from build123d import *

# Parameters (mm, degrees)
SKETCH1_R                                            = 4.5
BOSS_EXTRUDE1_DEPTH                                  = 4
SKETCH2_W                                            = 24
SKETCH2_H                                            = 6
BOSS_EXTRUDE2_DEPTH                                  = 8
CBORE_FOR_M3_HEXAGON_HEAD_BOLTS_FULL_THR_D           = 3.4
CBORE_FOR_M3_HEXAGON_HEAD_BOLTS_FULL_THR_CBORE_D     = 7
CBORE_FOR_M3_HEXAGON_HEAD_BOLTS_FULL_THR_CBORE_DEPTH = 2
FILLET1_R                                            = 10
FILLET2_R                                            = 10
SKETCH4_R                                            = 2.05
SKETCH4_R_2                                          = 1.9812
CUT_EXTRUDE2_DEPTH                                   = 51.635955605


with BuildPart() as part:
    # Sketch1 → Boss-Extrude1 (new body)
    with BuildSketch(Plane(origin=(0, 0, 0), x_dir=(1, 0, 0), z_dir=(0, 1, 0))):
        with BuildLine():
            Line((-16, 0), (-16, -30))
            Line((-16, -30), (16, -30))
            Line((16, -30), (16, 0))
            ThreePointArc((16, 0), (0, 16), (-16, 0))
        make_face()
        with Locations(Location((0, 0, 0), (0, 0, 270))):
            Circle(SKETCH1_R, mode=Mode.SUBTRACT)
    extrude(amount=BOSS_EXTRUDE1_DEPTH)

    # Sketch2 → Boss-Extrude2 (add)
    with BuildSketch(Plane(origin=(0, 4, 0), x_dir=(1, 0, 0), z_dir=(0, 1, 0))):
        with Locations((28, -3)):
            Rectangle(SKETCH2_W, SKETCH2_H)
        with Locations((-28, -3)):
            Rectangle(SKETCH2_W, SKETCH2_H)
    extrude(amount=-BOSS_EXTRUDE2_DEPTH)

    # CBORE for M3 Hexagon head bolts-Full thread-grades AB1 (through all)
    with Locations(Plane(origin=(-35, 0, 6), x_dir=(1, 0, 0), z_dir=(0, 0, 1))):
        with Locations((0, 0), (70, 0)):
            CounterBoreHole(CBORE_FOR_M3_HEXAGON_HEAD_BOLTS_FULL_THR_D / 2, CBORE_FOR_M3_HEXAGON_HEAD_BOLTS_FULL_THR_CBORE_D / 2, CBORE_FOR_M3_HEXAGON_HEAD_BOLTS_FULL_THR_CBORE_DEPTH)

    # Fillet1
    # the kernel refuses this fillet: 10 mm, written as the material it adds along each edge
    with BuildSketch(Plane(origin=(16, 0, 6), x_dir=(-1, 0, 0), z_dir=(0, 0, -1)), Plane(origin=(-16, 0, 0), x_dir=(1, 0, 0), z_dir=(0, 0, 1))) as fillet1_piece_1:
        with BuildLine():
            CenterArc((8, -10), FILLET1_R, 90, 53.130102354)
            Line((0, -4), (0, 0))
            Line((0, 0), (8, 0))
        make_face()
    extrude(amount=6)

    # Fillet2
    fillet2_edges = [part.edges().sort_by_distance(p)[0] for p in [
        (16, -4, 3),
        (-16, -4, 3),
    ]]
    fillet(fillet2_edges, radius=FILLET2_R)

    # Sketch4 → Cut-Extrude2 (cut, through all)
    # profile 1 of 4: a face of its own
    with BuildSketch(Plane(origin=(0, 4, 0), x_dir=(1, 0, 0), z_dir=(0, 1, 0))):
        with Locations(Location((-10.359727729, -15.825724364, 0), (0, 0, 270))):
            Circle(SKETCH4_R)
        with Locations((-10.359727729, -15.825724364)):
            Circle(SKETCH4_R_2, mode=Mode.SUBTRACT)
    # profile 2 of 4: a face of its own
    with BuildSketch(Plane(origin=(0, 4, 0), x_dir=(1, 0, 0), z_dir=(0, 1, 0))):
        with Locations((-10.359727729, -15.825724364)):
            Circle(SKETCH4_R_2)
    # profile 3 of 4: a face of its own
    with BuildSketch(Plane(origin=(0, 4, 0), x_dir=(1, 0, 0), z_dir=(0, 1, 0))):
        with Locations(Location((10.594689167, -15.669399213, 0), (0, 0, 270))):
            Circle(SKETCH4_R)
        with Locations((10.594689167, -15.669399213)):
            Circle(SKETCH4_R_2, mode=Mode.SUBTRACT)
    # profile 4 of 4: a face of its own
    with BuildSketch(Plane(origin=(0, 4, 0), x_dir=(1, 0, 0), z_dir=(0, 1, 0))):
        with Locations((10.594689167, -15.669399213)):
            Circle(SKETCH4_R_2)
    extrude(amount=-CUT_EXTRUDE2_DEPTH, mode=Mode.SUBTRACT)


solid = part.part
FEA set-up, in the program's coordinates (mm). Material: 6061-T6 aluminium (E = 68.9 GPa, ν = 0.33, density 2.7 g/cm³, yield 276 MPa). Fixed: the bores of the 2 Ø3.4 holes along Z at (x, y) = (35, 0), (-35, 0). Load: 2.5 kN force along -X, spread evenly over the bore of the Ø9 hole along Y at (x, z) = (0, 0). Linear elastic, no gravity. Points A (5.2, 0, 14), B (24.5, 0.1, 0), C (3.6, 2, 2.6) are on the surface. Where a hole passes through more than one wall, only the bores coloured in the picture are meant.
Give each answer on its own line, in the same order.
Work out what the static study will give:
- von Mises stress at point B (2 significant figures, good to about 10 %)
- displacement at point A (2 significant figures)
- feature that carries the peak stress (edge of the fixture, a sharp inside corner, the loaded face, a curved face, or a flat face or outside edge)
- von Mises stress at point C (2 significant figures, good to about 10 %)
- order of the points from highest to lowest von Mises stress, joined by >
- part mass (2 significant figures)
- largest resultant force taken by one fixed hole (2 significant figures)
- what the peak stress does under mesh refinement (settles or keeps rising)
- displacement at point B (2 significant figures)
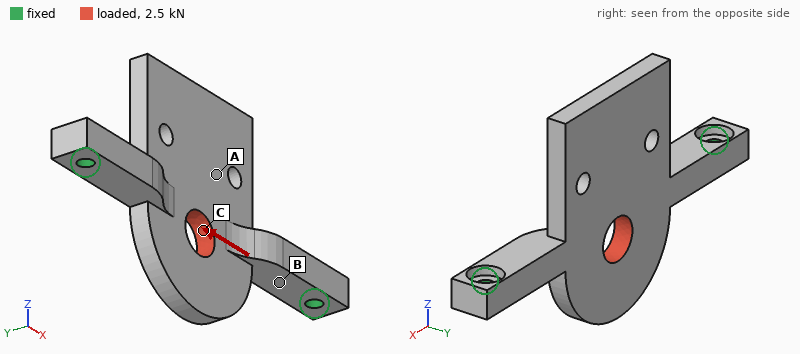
43 MPa
6.0 µm
edge of the fixture
32 MPa
B > C > A
20 g
1.3 kN
keeps rising
10 µm
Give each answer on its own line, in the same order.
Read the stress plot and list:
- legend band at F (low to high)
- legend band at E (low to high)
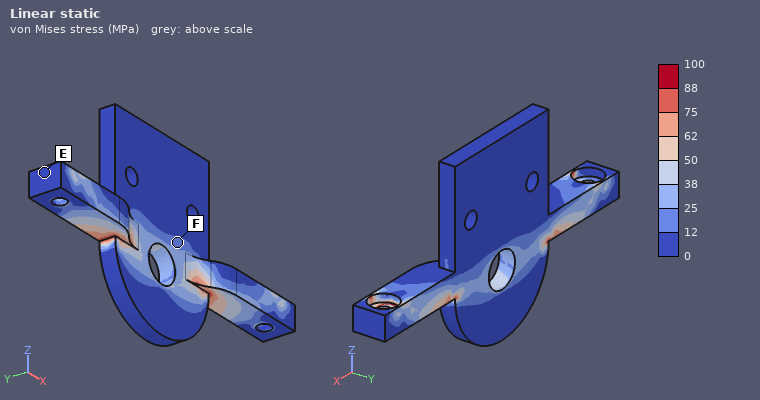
12 to 25 MPa
0 to 12 MPa
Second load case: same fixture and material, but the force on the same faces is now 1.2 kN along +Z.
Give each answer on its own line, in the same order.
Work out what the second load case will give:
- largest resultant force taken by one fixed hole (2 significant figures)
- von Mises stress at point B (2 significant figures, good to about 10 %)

660 N
32 MPa
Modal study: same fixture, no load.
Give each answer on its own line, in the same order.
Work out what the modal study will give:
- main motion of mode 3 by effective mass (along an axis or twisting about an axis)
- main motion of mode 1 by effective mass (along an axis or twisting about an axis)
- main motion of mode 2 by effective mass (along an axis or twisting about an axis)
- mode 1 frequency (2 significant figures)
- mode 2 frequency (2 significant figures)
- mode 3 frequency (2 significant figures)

along Z
along Y
along Y
2100 Hz
4000 Hz
4700 Hz
